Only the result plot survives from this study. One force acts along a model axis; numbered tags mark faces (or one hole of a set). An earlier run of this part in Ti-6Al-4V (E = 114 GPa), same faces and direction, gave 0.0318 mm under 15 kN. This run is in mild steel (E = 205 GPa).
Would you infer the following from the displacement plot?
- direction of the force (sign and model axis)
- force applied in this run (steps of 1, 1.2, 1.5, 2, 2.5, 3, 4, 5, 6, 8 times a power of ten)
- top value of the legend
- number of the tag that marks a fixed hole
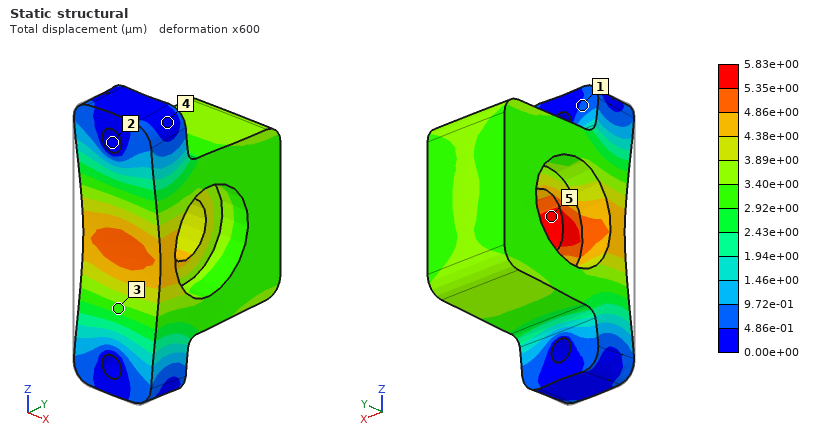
+Y
5 kN
5.83e+00 µm
2
